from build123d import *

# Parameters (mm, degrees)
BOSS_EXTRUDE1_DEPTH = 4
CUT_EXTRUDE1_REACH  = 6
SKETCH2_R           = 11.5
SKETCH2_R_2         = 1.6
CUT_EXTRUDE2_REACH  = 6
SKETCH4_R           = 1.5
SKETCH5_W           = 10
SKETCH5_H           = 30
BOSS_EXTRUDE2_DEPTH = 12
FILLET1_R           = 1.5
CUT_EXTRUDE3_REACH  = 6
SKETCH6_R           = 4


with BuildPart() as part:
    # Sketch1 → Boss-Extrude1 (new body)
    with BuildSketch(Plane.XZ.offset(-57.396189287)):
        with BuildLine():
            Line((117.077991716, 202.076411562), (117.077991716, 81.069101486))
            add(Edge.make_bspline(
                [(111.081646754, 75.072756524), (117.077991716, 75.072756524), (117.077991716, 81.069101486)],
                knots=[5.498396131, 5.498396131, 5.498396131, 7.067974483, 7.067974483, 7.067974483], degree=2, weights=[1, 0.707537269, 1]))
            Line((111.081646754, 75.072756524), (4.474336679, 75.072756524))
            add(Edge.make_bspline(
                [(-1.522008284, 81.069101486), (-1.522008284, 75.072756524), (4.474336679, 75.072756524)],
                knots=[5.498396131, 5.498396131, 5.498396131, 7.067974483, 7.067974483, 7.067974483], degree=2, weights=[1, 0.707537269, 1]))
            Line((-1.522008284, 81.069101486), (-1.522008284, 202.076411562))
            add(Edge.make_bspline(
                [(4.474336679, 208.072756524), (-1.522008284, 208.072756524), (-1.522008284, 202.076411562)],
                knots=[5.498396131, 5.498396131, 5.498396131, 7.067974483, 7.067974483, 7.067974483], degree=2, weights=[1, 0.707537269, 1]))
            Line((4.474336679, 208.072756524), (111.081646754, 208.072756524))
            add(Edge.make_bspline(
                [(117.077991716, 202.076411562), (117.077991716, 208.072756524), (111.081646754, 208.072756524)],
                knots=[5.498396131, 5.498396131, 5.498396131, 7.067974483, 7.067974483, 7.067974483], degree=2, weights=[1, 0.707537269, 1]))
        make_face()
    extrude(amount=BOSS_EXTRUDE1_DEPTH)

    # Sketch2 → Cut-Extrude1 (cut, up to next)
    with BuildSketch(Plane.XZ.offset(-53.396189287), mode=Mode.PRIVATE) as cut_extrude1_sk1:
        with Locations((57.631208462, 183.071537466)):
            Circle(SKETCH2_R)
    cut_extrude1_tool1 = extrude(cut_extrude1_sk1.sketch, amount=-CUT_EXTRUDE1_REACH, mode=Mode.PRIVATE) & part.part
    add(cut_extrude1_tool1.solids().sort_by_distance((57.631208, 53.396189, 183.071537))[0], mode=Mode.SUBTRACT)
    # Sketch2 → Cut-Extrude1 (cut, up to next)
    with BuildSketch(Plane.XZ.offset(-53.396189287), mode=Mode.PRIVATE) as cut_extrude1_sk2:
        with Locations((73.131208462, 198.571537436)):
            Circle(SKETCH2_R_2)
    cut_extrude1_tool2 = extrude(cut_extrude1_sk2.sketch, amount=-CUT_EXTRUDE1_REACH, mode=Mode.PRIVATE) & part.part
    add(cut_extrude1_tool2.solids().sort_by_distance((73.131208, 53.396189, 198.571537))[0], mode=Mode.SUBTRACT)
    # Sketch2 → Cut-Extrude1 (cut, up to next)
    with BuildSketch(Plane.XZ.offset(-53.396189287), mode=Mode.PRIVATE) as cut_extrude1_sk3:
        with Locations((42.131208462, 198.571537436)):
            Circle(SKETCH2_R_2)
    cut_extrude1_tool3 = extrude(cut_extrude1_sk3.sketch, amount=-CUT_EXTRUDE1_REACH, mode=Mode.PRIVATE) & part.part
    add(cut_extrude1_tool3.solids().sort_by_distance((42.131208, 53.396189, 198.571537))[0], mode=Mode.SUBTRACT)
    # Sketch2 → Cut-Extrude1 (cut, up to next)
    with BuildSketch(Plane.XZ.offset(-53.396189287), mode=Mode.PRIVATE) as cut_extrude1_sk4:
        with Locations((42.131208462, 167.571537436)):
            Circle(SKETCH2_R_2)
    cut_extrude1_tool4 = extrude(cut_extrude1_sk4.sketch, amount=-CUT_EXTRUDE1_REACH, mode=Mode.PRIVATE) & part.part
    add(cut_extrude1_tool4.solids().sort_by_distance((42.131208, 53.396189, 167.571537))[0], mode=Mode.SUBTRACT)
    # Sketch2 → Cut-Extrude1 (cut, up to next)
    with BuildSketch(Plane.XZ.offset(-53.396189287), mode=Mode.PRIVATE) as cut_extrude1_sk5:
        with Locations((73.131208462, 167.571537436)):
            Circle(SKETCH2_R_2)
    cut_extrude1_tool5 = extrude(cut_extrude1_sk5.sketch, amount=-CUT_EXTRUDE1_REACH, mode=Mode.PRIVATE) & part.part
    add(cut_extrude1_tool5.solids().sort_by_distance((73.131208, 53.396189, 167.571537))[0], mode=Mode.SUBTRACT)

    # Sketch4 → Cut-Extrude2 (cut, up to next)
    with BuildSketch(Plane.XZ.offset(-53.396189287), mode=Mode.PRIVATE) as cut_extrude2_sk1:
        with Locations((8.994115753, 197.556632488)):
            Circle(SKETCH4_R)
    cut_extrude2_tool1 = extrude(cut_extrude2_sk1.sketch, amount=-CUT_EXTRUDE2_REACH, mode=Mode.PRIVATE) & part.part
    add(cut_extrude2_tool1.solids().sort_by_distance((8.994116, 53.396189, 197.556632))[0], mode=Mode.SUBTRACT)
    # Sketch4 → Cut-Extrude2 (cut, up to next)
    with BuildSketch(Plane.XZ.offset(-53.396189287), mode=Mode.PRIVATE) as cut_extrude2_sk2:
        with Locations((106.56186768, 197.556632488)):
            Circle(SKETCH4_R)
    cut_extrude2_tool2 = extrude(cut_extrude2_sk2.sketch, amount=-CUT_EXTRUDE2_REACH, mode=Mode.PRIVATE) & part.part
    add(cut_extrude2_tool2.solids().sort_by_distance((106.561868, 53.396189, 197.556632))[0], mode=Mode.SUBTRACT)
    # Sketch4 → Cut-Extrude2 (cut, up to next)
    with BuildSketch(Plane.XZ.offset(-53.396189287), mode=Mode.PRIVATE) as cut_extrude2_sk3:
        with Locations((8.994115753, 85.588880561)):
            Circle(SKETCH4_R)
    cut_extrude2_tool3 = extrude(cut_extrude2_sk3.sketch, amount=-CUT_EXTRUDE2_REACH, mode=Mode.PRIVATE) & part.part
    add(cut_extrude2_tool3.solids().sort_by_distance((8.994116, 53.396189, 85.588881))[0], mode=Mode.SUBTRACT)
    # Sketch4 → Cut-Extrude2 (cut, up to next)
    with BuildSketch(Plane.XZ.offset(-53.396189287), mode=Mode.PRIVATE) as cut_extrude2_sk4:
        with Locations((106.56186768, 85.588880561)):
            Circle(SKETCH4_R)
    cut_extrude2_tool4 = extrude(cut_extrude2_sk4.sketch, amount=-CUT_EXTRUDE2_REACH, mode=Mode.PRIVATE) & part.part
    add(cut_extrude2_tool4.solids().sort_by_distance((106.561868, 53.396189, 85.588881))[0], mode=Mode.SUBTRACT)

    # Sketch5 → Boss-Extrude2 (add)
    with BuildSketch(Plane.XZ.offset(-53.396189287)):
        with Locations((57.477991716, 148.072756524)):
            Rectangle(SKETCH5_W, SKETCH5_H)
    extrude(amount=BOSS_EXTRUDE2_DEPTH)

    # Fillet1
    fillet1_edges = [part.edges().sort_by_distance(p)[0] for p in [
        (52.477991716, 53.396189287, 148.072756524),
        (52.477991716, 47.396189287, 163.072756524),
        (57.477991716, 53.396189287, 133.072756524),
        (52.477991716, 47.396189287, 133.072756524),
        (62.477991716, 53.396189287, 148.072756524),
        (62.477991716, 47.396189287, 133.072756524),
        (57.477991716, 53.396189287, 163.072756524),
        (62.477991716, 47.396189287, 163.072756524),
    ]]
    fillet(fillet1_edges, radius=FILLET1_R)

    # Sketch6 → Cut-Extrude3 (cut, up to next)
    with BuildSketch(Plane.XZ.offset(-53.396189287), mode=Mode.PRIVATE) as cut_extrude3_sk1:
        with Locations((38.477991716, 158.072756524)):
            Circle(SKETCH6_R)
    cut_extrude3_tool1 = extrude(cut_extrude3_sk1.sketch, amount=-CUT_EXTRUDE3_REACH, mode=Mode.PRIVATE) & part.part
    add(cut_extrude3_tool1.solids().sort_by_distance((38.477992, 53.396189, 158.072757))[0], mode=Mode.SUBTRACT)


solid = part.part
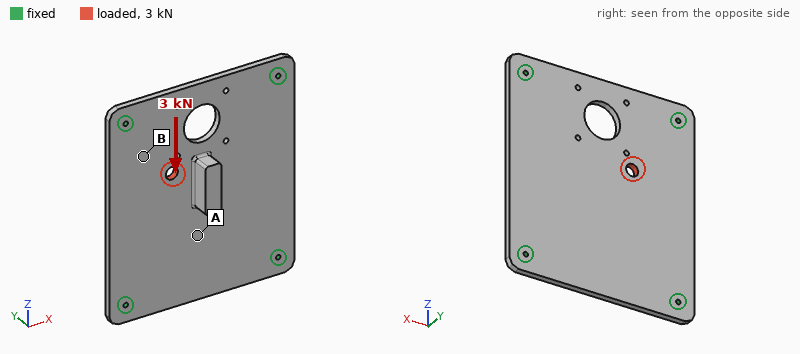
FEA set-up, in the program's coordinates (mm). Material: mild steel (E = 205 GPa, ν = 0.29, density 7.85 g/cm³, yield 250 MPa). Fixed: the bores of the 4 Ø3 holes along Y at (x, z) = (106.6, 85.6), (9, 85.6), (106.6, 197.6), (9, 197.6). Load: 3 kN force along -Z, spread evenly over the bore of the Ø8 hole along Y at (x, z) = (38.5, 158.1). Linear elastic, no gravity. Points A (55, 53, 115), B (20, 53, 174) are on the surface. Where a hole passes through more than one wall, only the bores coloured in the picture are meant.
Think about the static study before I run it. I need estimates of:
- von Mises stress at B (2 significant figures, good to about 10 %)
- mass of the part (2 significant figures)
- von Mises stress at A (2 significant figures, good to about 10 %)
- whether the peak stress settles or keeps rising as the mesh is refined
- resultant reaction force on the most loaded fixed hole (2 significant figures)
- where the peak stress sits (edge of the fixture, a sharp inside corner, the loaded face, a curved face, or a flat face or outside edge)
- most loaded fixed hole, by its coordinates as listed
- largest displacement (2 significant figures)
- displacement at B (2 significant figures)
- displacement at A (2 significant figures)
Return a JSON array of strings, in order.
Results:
["9.7 MPa", "510 g", "3.4 MPa", "keeps rising", "1.2 kN", "edge of the fixture", "(9, 197.6)", "4.8 µm", "2.1 µm", "1.9 µm"]
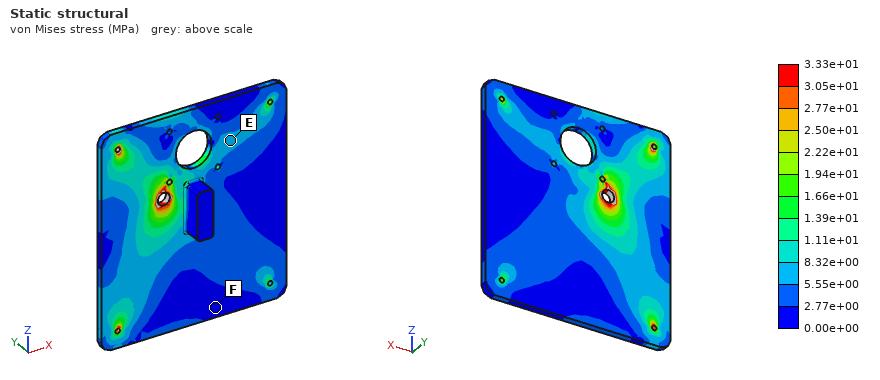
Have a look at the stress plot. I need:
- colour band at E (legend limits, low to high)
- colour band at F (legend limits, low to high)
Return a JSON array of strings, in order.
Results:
["5.55e+00 to 8.32e+00 MPa", "0.00e+00 to 2.77e+00 MPa"]
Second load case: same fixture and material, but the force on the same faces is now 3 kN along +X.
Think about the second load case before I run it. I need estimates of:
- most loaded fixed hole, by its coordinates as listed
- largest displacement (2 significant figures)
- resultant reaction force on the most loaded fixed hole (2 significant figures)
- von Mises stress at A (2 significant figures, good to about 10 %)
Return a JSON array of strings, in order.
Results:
["(9, 197.6)", "5.6 µm", "1.1 kN", "5.1 MPa"]
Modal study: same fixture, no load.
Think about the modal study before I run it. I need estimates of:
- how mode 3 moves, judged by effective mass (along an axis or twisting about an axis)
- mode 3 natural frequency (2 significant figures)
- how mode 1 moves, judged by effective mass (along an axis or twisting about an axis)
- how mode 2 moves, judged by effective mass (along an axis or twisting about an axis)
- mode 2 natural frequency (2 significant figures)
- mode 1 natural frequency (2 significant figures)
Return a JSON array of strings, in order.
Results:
["twisting about X", "2100 Hz", "along Y", "twisting about Z", "1800 Hz", "1100 Hz"]
